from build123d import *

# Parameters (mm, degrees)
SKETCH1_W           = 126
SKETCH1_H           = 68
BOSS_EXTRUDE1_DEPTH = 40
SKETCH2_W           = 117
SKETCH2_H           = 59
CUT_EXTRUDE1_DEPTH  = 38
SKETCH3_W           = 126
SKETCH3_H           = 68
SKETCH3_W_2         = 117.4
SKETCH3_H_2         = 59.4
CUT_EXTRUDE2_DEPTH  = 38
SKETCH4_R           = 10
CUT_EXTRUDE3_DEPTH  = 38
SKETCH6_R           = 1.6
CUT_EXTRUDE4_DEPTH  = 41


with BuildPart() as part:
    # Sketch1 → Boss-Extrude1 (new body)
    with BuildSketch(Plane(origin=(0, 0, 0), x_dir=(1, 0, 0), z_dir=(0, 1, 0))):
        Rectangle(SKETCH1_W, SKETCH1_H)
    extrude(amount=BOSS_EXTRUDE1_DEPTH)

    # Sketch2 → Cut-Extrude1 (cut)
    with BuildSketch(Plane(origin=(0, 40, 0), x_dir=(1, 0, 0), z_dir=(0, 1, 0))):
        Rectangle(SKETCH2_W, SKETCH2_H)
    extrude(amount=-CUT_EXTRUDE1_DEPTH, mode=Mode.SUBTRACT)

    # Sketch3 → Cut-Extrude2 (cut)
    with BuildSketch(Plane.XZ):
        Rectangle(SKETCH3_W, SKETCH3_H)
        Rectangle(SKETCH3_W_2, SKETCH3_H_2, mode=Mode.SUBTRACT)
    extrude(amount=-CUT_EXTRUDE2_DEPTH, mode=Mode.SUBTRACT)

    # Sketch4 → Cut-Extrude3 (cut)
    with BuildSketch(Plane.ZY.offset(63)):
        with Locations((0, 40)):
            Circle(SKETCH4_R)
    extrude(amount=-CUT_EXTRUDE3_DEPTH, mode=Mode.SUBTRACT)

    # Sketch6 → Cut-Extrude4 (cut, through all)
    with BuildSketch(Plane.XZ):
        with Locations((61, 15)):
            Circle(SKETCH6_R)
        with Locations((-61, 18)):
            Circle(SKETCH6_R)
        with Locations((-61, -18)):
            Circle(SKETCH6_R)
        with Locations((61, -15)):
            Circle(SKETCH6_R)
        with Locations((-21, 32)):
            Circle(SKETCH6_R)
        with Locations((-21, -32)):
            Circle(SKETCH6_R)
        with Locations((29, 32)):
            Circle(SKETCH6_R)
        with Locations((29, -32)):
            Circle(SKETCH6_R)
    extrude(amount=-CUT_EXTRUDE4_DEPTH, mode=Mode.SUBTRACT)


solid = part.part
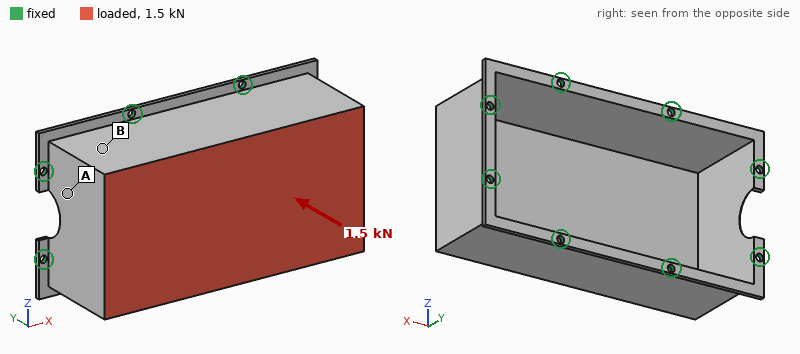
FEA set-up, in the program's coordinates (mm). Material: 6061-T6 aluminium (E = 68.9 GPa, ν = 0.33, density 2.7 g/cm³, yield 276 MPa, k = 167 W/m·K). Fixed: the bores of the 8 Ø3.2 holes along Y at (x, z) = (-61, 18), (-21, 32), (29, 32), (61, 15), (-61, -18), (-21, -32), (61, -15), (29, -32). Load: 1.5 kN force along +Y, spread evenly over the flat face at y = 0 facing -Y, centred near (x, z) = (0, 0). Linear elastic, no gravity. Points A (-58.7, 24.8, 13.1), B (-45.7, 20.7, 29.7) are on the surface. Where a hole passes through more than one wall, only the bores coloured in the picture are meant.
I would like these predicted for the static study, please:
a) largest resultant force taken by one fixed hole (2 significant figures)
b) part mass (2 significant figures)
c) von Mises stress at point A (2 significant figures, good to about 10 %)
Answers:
250 N
53 g
39 MPa
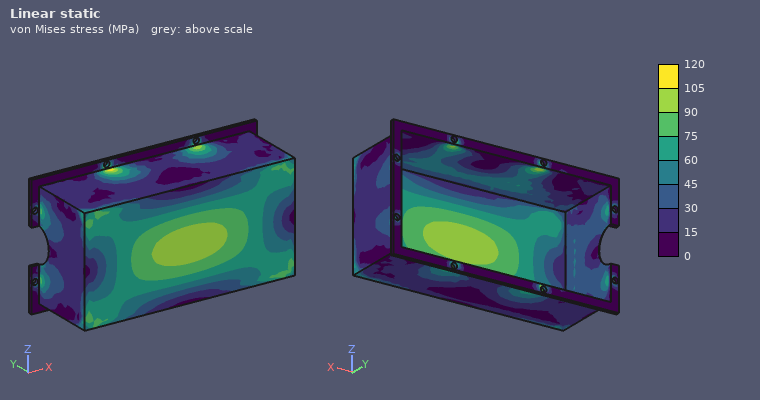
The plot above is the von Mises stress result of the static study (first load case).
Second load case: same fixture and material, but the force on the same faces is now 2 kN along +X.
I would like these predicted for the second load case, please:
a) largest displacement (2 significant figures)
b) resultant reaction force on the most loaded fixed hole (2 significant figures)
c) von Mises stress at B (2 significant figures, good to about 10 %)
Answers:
90 µm
520 N
67 MPa
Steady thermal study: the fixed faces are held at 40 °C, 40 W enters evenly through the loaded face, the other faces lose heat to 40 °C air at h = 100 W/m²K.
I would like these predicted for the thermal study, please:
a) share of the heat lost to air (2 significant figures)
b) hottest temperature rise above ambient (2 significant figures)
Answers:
95 %
28 K
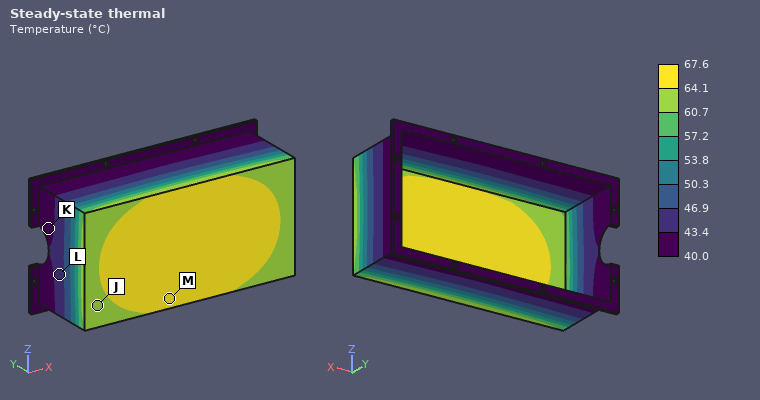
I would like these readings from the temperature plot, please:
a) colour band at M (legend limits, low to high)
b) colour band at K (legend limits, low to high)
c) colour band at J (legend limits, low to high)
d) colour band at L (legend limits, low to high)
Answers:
64.1 to 67.6 °C
40.0 to 43.4 °C
60.7 to 64.1 °C
43.4 to 46.9 °C
